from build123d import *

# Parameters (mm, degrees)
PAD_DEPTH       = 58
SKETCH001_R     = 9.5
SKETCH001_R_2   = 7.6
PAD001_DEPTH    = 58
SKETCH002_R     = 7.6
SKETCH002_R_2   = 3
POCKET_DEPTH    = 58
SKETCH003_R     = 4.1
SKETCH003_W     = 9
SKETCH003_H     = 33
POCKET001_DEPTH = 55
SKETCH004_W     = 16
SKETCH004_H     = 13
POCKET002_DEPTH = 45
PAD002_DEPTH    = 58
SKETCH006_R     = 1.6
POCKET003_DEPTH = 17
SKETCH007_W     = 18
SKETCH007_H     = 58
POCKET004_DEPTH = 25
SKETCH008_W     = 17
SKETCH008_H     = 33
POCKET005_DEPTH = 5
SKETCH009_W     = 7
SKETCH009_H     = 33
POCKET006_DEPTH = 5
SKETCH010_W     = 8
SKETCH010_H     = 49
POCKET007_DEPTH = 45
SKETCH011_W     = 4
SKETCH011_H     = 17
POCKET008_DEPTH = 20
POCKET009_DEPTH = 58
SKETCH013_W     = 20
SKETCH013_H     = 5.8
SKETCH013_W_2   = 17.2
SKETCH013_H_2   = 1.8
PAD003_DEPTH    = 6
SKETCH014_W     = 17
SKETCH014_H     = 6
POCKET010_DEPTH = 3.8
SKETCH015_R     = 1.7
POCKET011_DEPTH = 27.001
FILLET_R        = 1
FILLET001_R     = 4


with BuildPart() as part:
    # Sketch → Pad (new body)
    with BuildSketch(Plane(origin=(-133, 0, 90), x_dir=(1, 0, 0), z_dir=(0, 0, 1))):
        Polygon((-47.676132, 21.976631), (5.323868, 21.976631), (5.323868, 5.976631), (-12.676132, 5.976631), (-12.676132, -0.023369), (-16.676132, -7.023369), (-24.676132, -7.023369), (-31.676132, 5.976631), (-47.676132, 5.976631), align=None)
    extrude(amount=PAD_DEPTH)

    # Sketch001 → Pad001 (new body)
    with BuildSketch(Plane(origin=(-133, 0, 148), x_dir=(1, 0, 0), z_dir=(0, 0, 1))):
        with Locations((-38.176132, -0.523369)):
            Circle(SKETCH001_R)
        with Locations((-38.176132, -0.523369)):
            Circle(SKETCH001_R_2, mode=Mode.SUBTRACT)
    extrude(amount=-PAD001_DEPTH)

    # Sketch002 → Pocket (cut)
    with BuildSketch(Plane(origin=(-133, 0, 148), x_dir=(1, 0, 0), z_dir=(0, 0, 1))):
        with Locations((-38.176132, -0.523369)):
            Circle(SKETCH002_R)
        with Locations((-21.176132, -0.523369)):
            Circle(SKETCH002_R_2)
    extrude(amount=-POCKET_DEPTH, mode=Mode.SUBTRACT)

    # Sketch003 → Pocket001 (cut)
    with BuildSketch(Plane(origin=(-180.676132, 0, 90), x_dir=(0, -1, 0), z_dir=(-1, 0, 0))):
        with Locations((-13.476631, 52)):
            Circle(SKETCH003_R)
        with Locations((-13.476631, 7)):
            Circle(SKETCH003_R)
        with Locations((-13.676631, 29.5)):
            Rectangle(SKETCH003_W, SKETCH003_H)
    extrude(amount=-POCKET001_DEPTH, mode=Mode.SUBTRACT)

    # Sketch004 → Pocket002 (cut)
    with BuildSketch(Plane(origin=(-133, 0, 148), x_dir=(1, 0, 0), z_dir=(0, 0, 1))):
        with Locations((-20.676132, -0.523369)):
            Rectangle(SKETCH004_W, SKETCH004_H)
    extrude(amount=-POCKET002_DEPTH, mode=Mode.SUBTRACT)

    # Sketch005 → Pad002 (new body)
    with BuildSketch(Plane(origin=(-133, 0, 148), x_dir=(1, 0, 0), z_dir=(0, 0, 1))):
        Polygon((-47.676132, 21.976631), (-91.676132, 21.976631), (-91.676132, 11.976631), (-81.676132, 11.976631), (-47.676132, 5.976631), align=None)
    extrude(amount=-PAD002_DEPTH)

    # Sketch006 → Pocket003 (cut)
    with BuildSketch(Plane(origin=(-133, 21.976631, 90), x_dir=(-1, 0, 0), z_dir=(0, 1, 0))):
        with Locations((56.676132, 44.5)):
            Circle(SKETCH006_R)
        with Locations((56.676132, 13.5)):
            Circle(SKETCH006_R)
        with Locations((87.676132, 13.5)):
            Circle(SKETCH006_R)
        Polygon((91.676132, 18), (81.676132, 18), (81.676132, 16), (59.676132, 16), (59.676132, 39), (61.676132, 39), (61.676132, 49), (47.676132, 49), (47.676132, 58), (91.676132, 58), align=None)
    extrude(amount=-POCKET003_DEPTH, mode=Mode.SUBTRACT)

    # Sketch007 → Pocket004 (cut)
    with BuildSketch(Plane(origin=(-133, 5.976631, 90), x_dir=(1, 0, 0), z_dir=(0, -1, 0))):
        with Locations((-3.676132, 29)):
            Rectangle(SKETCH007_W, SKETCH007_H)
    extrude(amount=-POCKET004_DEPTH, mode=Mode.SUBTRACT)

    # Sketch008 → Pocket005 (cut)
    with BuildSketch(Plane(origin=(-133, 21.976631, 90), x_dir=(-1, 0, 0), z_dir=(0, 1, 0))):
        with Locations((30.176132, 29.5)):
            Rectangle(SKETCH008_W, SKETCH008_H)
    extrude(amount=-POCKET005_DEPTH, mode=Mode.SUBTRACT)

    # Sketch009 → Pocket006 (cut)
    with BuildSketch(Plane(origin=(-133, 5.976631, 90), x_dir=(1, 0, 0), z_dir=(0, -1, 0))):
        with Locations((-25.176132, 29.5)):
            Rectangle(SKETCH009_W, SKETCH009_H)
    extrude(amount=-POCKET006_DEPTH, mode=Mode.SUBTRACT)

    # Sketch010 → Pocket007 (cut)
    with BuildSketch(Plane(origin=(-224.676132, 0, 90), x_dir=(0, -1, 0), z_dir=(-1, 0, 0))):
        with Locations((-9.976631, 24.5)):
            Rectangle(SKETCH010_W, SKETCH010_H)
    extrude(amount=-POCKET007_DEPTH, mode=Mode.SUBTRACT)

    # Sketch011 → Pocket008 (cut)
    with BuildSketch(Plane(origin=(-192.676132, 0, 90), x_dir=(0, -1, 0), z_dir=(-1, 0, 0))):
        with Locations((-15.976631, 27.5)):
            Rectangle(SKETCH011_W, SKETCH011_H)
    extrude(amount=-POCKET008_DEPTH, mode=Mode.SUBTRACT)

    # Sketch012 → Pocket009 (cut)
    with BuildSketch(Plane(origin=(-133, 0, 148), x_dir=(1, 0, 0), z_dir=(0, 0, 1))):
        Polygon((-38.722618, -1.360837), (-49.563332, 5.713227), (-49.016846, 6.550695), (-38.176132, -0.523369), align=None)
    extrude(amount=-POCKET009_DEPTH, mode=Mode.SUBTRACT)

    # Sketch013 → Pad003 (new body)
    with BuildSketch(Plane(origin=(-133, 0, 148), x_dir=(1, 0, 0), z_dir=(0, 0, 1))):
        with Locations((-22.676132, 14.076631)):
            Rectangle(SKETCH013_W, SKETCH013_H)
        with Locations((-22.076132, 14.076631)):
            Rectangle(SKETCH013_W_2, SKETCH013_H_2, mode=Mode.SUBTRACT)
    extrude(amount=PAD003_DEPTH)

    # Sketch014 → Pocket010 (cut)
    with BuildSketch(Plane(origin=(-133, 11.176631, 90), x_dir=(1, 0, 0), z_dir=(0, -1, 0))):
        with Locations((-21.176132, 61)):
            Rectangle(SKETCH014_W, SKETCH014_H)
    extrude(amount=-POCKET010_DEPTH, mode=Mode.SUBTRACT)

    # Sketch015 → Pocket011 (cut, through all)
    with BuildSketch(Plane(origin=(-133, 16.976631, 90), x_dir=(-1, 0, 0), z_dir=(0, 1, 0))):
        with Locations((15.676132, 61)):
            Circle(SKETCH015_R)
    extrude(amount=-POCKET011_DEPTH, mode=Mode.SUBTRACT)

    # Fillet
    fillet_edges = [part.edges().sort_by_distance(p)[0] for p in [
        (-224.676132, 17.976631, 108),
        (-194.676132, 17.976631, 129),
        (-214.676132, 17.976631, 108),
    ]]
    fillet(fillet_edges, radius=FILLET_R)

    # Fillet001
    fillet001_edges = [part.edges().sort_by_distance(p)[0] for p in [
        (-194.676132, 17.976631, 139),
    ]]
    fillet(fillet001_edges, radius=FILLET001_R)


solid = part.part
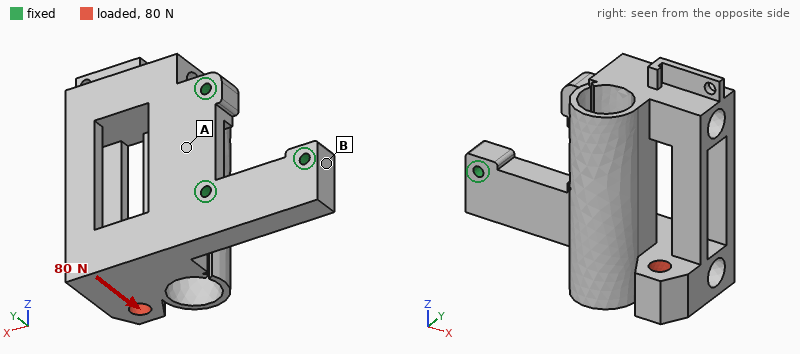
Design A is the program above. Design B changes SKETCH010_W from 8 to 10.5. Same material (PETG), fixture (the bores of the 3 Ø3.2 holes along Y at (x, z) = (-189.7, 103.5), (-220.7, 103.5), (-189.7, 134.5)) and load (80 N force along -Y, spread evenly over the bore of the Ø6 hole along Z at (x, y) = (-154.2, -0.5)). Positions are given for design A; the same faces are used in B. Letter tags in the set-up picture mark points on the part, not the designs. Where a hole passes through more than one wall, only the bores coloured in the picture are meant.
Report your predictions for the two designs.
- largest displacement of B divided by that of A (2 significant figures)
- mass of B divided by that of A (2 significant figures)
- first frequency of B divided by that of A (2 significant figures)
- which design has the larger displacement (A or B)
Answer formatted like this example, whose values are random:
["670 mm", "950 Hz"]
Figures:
["1.4", "0.96", "0.84", "B"]
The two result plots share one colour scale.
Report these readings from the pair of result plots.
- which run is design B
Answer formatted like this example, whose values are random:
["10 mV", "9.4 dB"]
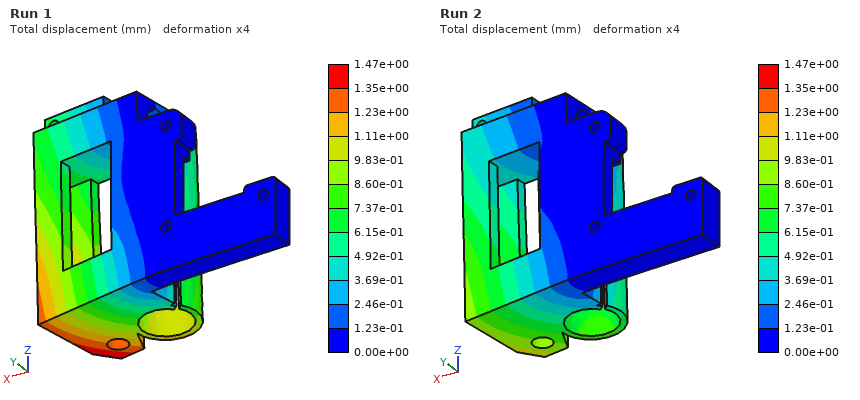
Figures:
["Run 1"]
